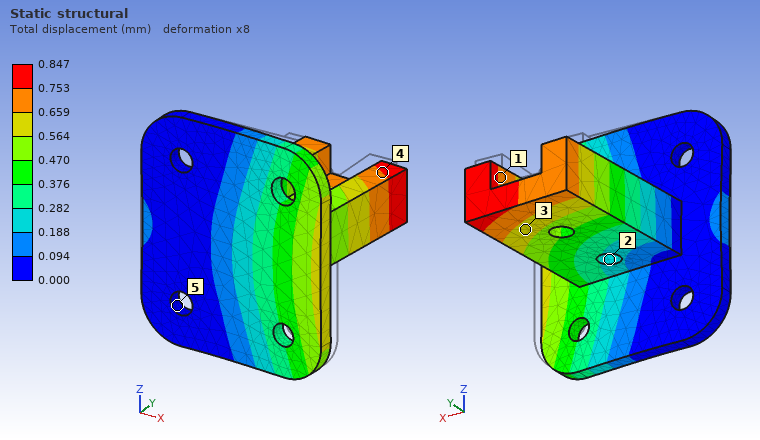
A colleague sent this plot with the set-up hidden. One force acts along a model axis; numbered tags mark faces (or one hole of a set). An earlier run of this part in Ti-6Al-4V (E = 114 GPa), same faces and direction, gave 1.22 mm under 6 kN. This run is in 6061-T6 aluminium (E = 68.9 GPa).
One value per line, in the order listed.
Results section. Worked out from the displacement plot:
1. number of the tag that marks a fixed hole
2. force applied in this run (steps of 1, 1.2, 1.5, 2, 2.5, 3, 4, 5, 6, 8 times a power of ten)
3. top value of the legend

5
2.5 kN
0.847 mm
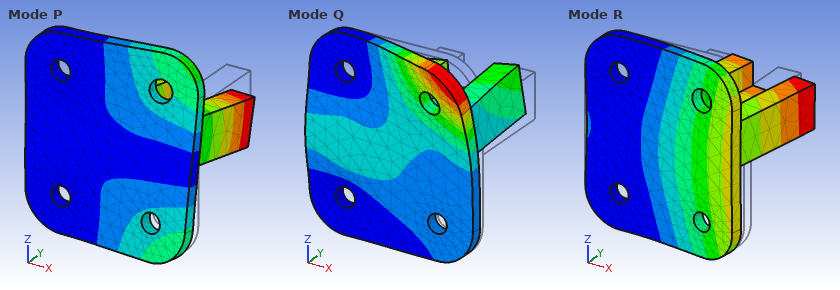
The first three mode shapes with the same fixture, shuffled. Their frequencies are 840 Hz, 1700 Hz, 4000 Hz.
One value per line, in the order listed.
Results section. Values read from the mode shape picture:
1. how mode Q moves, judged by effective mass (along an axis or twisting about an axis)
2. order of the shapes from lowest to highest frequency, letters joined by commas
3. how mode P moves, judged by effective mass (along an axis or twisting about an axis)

along Y
R, P, Q
along Z
